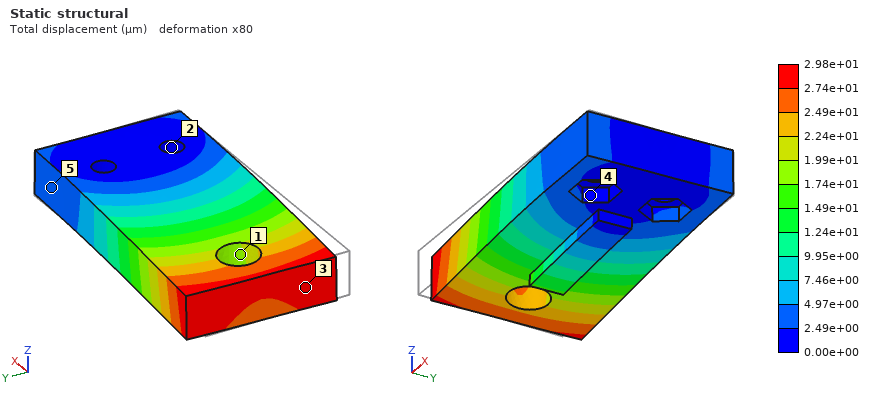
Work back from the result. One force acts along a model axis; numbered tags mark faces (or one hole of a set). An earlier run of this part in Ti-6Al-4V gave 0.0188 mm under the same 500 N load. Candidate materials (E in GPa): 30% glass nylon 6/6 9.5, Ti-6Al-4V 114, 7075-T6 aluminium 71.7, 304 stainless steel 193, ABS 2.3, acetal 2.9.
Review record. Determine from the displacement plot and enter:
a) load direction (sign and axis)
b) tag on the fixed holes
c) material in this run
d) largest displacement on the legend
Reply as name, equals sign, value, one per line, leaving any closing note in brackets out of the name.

load direction = +Y
tag on the fixed holes = 2
material in this run = 7075-T6 aluminium
largest displacement on the legend = 2.98e+01 µm
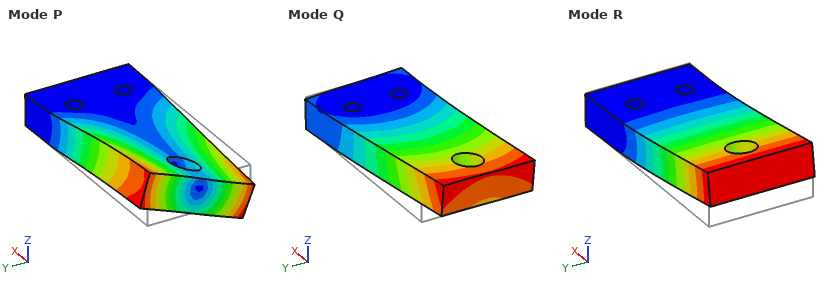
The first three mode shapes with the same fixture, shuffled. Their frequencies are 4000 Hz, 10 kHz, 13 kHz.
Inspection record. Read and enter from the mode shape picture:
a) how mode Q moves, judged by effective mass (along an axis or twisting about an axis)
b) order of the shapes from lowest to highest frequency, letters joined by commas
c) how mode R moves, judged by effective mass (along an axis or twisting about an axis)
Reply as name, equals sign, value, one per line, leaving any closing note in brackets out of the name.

how mode Q moves, judged by effective mass = along Y
order of the shapes from lowest to highest frequency, letters joined by commas = R, Q, P
how mode R moves, judged by effective mass = along Z
